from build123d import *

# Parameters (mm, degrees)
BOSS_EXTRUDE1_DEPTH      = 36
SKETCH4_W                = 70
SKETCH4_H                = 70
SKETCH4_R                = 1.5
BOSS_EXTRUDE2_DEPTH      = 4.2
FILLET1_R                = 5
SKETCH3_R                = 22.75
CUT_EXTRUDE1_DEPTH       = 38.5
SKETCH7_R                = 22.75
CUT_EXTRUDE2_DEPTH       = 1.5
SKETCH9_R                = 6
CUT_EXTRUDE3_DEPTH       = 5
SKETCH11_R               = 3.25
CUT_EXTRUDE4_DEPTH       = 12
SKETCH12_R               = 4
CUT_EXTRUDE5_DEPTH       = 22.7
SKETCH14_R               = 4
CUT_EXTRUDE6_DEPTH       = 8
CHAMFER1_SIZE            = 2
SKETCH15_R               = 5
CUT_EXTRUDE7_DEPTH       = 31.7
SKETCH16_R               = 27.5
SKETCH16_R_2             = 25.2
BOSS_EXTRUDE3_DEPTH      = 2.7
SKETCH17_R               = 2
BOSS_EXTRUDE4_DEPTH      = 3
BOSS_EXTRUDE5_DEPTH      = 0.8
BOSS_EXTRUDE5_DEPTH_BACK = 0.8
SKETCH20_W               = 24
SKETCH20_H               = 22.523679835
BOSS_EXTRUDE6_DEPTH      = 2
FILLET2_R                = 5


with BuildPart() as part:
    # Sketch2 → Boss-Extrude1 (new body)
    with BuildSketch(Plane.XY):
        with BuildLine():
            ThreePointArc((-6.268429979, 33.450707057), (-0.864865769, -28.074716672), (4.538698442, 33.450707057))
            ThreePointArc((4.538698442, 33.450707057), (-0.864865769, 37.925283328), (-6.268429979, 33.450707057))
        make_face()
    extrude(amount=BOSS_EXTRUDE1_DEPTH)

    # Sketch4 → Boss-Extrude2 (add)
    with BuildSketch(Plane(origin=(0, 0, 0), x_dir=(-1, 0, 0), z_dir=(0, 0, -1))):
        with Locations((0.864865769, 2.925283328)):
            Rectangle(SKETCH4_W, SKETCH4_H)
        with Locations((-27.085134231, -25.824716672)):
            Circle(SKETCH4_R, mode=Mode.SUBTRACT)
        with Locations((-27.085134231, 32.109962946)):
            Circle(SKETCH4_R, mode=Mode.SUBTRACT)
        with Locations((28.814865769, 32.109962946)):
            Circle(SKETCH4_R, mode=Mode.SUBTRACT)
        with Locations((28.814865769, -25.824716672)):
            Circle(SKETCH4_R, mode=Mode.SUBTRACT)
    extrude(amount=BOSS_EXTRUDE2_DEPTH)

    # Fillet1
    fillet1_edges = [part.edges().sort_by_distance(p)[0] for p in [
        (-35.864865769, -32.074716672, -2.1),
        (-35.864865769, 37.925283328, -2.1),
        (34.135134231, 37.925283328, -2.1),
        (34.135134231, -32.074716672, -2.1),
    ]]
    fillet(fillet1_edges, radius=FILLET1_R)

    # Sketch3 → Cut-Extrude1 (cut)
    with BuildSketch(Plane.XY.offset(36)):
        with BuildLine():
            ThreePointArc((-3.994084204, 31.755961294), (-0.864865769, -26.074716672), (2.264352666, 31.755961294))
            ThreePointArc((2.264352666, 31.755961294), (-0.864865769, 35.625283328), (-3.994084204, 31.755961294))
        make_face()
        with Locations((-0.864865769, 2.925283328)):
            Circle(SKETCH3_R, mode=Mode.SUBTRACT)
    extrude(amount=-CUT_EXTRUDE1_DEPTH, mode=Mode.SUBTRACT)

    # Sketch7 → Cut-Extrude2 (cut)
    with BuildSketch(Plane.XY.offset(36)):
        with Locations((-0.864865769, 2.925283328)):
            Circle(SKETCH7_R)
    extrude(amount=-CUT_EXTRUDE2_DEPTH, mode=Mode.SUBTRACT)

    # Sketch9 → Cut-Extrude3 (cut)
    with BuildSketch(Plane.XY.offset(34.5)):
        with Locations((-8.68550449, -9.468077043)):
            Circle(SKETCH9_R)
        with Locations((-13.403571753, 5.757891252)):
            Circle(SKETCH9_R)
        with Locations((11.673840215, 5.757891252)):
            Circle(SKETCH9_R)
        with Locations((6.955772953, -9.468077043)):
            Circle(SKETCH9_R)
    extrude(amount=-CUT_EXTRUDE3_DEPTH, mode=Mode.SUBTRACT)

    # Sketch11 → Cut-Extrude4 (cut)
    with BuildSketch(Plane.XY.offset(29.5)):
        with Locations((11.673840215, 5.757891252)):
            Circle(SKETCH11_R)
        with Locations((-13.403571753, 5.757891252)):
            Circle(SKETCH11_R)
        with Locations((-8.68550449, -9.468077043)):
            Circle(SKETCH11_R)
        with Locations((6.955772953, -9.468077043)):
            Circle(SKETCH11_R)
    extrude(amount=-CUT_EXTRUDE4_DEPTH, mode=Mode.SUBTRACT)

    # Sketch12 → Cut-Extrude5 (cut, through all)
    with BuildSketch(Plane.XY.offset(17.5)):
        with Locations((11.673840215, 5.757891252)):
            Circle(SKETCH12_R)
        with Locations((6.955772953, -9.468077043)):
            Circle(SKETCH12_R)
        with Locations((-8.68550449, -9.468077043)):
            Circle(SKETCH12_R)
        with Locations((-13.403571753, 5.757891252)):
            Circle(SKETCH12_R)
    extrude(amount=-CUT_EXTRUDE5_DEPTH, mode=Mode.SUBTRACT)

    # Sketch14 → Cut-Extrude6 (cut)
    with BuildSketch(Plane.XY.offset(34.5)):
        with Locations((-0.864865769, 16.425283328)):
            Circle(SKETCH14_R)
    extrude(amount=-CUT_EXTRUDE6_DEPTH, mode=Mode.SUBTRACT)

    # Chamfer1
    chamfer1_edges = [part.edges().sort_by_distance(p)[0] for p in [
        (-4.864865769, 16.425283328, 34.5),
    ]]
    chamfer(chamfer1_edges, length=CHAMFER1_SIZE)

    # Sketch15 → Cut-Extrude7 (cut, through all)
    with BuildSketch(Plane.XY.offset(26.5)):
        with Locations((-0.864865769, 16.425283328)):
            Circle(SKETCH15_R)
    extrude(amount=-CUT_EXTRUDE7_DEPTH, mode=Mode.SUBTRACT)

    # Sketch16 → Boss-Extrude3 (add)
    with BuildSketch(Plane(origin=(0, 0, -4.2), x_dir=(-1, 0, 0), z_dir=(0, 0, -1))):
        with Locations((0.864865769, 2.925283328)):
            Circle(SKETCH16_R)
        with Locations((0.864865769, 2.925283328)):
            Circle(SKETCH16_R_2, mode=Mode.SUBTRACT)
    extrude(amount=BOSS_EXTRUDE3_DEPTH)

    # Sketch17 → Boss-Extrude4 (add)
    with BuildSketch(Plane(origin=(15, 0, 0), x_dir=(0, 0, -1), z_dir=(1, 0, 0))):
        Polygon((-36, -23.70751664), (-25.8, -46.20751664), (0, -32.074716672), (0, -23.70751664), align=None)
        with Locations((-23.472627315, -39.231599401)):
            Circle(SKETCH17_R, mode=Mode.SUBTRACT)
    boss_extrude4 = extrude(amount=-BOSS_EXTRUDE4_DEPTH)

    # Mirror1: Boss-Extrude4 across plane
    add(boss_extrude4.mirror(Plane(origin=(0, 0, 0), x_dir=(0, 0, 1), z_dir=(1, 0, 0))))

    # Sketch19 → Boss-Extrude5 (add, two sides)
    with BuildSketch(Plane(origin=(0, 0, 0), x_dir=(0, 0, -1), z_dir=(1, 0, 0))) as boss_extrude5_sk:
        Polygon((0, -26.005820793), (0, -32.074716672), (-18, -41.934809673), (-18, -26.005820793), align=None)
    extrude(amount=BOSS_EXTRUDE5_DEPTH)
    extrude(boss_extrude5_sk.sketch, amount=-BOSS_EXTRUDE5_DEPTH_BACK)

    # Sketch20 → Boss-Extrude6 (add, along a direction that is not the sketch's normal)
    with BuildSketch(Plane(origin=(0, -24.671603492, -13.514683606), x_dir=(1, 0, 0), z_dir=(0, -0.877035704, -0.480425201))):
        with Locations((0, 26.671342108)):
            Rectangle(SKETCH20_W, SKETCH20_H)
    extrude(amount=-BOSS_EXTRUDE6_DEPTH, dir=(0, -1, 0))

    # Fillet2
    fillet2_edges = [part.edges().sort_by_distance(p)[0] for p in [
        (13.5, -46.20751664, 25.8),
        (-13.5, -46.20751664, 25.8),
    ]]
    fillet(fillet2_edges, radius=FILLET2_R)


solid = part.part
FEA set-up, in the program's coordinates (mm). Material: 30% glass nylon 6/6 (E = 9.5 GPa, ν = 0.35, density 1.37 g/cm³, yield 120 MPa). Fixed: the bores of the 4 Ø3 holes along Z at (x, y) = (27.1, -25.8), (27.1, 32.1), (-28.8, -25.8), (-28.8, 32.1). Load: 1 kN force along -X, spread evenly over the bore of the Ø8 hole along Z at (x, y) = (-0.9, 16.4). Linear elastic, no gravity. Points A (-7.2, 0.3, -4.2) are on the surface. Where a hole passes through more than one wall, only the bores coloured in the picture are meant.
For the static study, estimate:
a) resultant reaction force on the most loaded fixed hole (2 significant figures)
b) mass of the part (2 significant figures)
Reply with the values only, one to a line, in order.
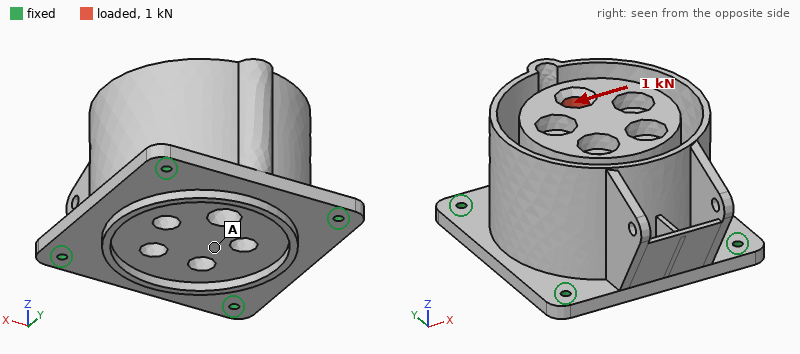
440 N
110 g
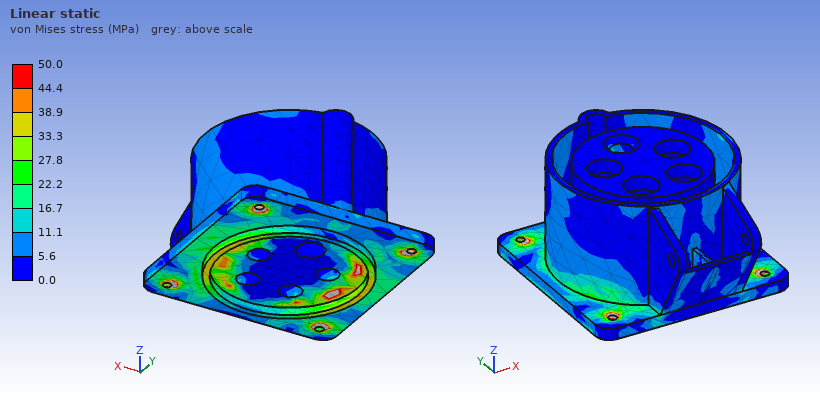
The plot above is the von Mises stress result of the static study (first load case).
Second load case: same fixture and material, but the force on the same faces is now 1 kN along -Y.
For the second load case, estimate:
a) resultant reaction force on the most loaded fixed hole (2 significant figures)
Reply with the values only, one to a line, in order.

430 N
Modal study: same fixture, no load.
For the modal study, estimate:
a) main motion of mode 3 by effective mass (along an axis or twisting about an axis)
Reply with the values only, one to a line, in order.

along Z
